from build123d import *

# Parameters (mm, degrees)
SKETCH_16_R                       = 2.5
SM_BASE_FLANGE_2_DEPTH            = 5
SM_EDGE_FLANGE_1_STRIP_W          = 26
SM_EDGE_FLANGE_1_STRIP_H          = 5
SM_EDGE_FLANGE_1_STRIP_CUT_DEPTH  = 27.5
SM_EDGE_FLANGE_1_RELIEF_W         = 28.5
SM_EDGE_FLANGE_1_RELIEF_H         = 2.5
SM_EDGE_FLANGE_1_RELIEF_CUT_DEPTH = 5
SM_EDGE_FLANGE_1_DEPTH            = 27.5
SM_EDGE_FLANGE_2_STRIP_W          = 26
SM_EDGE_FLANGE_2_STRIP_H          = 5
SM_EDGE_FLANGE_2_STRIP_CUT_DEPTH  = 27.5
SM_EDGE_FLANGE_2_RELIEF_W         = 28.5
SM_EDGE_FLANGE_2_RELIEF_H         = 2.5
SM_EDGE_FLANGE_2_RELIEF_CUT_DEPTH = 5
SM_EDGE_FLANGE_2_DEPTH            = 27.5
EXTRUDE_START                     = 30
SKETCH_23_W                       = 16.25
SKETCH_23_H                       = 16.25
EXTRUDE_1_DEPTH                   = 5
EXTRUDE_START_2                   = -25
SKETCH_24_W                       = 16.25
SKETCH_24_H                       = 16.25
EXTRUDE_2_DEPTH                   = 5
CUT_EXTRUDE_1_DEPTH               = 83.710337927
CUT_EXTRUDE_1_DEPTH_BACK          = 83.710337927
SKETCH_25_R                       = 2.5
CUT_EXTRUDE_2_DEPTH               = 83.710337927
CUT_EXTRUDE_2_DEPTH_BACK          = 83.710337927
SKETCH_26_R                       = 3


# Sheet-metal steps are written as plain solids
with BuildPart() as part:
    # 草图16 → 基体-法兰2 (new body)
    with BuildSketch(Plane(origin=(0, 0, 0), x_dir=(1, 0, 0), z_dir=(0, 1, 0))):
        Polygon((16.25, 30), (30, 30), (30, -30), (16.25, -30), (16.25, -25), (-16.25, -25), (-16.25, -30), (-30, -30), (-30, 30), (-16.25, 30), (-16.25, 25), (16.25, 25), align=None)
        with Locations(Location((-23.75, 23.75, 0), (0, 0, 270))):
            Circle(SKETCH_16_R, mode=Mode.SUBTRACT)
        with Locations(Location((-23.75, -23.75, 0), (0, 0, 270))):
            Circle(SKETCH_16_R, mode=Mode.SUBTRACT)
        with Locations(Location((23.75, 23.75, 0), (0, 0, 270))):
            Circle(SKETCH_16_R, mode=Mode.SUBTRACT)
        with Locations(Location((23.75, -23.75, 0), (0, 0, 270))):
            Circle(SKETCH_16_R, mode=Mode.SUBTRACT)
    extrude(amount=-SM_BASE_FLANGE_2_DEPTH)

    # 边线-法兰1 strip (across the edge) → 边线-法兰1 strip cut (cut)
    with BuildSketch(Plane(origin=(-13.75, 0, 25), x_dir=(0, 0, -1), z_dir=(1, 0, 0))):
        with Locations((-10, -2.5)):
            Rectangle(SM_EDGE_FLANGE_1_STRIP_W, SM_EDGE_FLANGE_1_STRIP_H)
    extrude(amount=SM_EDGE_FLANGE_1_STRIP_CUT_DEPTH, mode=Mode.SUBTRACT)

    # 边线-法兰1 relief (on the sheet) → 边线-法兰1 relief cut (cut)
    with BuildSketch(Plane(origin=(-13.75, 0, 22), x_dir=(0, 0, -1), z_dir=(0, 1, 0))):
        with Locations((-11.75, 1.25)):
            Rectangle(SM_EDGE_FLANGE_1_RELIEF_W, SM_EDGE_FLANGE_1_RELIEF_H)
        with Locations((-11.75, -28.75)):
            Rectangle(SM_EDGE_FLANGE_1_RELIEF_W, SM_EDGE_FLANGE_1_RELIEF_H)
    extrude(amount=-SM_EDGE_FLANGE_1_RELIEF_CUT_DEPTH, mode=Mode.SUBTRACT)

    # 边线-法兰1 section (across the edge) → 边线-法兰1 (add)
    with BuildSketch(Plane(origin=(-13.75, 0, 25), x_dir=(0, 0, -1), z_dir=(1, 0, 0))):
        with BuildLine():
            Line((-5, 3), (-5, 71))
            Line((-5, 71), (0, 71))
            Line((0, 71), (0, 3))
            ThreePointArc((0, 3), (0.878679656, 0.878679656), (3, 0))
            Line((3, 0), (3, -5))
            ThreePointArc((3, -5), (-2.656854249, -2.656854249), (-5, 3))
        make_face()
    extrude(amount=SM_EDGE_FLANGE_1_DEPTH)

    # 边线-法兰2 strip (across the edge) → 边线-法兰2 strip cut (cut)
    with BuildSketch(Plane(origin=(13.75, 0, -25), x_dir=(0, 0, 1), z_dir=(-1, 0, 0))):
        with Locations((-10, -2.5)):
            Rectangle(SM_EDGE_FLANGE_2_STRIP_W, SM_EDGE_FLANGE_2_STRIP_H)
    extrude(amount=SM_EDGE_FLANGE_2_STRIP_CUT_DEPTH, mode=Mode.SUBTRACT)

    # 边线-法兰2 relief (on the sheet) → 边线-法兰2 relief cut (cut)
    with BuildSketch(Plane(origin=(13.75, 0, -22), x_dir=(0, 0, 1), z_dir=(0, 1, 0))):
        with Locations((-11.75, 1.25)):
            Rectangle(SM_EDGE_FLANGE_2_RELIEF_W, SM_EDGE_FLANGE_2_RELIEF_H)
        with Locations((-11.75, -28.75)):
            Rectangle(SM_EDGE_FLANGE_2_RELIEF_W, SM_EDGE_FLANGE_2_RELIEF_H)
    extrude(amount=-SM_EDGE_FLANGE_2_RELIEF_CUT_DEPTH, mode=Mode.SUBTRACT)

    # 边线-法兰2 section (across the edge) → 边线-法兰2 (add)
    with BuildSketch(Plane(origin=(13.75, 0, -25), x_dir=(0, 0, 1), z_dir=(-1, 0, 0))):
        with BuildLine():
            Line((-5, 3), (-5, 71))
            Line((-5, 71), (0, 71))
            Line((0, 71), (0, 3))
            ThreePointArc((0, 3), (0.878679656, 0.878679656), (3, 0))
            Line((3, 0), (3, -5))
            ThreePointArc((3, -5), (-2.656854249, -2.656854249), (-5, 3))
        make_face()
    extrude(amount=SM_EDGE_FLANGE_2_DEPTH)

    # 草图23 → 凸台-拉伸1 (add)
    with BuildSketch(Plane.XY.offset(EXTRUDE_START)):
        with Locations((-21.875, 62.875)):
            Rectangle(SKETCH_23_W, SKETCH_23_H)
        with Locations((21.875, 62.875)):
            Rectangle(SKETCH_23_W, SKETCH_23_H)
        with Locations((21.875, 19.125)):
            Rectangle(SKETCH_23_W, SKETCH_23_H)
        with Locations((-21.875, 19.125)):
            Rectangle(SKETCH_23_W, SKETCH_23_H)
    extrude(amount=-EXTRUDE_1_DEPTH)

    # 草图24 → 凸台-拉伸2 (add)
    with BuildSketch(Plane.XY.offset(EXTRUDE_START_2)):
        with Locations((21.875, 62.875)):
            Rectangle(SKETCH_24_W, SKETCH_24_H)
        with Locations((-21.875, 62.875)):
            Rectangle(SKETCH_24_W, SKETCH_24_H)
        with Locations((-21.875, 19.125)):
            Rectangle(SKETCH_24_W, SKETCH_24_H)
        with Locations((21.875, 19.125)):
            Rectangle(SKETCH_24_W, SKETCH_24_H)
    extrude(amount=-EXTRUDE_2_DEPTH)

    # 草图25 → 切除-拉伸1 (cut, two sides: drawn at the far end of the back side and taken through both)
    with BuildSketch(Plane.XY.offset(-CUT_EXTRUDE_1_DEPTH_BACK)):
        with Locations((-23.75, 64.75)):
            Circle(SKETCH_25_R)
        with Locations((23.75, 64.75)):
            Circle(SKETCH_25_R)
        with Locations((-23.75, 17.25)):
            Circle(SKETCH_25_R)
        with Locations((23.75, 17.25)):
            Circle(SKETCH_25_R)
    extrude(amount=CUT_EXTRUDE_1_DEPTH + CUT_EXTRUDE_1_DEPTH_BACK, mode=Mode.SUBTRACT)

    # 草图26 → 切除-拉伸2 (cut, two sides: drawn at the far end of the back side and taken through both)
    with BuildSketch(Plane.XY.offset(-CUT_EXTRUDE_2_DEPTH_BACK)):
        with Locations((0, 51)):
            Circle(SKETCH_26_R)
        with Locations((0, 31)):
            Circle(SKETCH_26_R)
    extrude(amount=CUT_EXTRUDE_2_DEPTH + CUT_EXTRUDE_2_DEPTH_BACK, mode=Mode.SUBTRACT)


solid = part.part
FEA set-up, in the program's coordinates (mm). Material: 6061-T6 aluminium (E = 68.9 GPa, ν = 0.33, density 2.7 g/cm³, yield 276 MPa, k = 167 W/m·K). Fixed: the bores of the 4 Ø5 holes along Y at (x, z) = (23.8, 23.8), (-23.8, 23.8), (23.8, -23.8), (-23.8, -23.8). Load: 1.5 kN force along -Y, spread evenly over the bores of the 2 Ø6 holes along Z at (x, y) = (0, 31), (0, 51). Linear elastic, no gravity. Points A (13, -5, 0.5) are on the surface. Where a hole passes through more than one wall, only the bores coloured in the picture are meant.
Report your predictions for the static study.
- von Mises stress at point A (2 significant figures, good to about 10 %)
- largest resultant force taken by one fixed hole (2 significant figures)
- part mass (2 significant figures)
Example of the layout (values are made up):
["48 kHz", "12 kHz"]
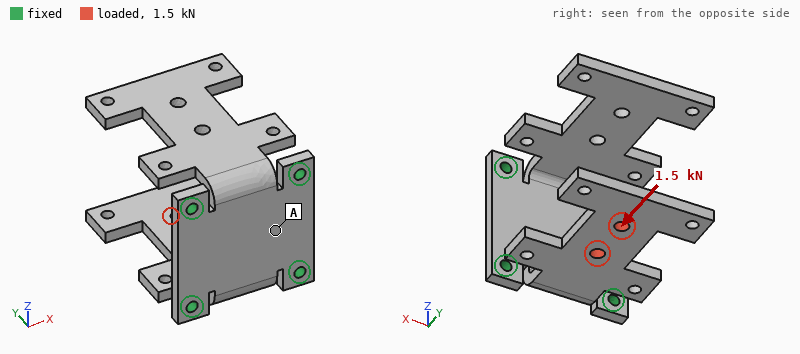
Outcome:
["24 MPa", "890 N", "120 g"]
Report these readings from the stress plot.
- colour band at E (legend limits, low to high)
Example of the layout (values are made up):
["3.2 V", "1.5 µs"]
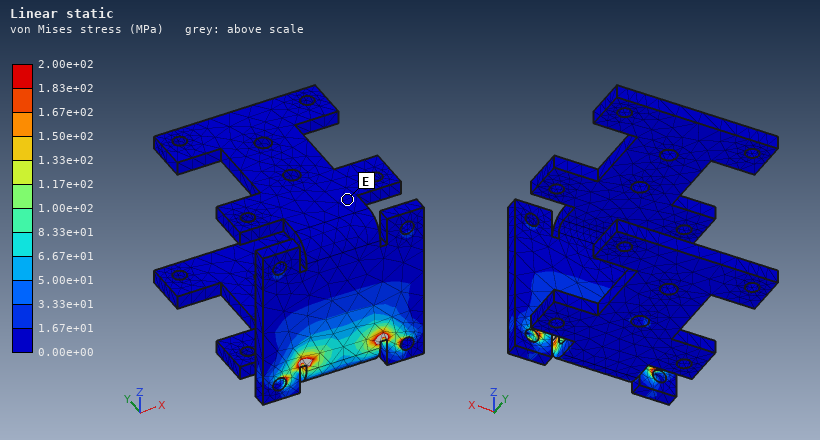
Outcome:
["0.00e+00 to 1.67e+01 MPa"]
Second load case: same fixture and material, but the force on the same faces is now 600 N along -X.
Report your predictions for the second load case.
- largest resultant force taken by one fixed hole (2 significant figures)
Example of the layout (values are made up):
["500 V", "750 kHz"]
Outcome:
["770 N"]
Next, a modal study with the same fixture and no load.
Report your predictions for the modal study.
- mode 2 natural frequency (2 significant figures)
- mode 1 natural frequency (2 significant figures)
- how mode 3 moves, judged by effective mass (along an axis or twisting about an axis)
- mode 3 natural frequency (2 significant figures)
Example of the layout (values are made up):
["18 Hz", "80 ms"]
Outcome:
["450 Hz", "440 Hz", "along X", "1000 Hz"]
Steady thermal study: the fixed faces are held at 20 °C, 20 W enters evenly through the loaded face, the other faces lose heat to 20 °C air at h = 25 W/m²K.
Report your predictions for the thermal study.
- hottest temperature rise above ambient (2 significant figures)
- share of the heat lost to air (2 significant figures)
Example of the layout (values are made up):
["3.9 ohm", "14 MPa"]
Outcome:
["40 K", "34 %"]
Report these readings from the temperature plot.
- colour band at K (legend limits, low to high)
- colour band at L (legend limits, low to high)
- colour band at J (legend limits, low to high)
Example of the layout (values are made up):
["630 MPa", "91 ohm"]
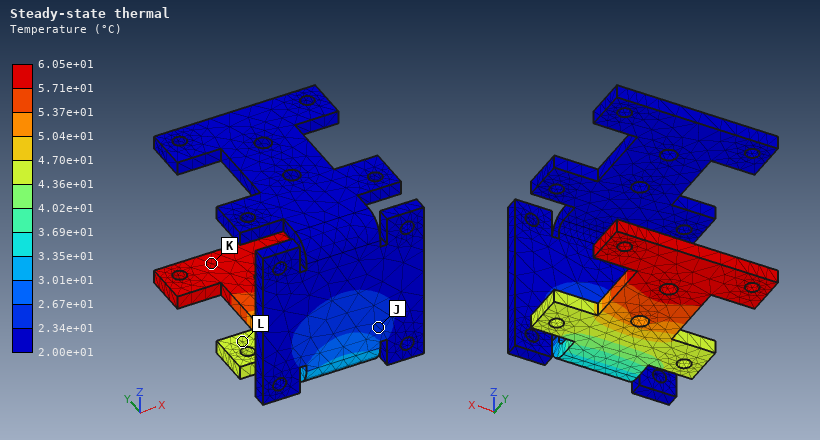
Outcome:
["5.71e+01 to 6.05e+01 °C", "4.36e+01 to 4.70e+01 °C", "2.34e+01 to 2.67e+01 °C"]
